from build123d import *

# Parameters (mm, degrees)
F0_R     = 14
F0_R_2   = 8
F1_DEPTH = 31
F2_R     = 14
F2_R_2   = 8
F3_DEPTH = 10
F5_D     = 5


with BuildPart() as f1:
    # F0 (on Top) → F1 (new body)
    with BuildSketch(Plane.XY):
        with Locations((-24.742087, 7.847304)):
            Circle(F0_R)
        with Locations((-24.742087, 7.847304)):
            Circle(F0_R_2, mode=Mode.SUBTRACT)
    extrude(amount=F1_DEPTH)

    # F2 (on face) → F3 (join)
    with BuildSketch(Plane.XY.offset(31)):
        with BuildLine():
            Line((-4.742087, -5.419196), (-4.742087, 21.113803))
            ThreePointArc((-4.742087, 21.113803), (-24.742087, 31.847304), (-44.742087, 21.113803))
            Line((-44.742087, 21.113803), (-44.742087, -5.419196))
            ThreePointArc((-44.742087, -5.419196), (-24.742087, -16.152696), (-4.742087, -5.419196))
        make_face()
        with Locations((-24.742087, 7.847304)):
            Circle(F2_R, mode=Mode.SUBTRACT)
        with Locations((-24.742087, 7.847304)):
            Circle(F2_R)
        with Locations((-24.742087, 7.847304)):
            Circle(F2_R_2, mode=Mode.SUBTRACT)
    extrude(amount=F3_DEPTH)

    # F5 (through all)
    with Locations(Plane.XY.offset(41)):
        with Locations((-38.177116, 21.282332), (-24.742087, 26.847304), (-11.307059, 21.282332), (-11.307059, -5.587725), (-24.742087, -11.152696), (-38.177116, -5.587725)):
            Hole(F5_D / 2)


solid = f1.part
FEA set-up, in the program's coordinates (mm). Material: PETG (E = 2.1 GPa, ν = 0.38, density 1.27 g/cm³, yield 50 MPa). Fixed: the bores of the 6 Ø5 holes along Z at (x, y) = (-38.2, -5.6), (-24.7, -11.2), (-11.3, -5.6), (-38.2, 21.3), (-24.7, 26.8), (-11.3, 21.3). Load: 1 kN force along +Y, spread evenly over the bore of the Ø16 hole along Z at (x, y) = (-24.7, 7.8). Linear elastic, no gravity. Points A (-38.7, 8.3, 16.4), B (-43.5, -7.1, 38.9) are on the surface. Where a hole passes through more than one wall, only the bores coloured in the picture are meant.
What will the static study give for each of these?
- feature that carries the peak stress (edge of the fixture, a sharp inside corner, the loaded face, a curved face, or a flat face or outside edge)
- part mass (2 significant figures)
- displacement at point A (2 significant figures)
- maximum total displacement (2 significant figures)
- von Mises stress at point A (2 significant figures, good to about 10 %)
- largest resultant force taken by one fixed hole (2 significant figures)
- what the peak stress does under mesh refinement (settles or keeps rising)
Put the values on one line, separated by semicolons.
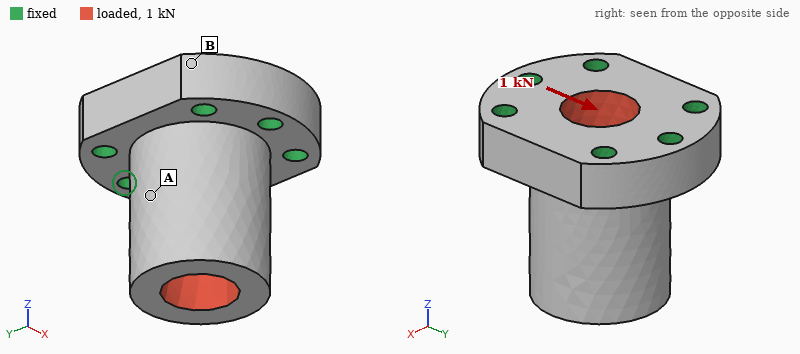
a sharp inside corner; 33 g; 0.078 mm; 0.16 mm; 2.6 MPa; 310 N; keeps rising
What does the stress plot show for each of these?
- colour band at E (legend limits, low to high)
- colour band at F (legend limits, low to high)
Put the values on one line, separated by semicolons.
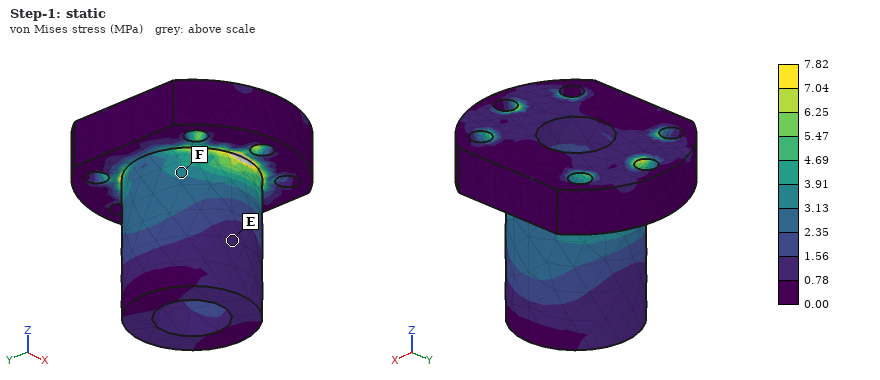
0.78 to 1.56 MPa; 3.13 to 3.91 MPa
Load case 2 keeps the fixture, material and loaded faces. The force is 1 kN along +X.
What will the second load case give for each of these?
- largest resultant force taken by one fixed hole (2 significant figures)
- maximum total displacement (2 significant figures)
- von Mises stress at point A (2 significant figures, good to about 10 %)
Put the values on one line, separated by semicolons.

360 N; 0.20 mm; 1.6 MPa
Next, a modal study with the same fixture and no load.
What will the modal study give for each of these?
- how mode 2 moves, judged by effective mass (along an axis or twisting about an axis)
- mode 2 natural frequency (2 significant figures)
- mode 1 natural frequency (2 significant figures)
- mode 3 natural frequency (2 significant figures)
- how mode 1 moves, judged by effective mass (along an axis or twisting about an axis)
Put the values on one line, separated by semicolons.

along Y; 3200 Hz; 2900 Hz; 5600 Hz; along X
